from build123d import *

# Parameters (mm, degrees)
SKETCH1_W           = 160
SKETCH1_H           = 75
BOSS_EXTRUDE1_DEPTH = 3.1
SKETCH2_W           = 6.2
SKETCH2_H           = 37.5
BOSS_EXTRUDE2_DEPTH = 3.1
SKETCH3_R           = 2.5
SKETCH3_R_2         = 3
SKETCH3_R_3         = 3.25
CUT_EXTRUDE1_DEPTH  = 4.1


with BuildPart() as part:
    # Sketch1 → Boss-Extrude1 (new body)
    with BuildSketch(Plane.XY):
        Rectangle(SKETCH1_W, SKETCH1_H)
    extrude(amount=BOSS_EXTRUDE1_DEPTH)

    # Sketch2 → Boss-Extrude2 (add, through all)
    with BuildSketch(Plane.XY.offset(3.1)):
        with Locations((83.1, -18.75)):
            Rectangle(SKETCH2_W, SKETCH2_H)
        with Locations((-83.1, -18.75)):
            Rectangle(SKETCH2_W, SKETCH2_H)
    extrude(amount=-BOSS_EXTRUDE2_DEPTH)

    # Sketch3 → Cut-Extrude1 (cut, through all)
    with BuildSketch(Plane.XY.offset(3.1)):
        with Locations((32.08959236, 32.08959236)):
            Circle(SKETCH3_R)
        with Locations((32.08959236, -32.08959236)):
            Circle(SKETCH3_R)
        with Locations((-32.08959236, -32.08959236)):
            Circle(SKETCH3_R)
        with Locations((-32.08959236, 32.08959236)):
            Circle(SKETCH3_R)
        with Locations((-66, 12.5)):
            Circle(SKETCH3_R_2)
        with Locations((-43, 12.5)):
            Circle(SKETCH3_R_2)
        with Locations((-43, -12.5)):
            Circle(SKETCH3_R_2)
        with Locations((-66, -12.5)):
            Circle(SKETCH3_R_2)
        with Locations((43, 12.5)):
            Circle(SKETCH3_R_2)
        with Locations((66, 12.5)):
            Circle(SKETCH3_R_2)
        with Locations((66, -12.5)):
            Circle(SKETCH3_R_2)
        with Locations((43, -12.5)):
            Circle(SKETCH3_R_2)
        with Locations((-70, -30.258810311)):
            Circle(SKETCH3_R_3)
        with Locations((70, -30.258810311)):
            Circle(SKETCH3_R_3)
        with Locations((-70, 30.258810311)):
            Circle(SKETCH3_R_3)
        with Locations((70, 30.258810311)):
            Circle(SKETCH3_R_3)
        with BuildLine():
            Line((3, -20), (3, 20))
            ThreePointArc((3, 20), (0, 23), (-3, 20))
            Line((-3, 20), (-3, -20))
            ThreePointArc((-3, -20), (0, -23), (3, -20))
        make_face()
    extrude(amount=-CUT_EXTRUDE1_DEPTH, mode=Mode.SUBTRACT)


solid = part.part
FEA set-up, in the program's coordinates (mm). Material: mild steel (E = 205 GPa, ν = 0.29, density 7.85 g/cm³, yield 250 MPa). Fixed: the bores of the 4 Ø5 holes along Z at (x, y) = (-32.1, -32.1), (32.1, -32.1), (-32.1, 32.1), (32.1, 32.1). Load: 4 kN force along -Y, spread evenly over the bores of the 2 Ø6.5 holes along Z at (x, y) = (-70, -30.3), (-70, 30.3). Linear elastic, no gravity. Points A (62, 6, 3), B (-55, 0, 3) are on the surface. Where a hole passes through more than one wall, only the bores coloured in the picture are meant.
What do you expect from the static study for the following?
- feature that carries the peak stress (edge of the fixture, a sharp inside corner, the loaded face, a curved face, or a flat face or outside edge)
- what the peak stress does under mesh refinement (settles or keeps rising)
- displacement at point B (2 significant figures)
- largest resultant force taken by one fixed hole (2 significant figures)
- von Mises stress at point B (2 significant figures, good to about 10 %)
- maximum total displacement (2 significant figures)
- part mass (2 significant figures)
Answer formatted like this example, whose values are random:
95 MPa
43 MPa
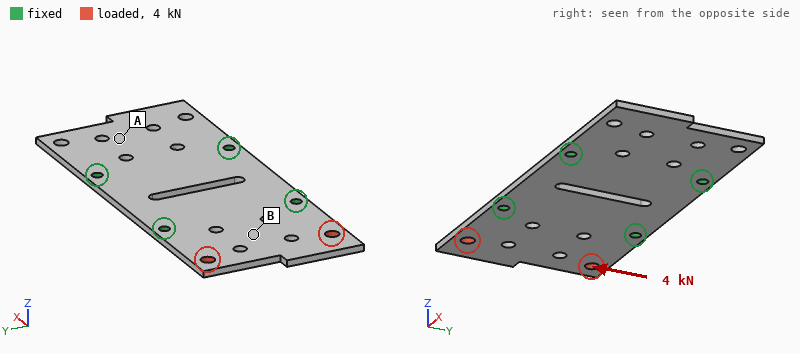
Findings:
edge of the fixture
keeps rising
8.9 µm
3.0 kN
29 MPa
20 µm
290 g
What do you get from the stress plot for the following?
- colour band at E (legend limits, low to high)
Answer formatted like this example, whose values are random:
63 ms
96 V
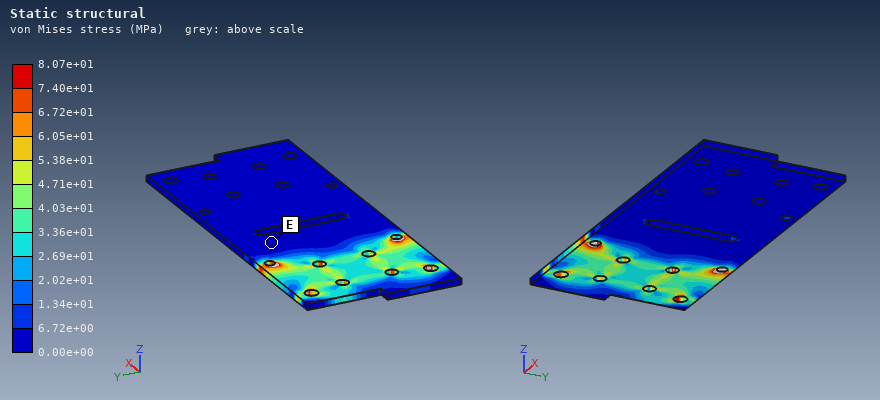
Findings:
0.00e+00 to 6.72e+00 MPa
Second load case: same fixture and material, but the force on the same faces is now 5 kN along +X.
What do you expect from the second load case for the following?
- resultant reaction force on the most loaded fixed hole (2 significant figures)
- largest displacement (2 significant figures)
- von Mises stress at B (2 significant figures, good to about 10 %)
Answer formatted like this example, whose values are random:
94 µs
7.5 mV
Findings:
2.3 kN
10 µm
7.7 MPa
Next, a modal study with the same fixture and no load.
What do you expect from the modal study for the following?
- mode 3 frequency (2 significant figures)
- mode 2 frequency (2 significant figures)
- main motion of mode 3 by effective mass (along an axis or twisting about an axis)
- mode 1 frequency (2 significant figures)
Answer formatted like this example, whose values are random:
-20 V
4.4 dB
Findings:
1900 Hz
860 Hz
twisting about X
840 Hz
